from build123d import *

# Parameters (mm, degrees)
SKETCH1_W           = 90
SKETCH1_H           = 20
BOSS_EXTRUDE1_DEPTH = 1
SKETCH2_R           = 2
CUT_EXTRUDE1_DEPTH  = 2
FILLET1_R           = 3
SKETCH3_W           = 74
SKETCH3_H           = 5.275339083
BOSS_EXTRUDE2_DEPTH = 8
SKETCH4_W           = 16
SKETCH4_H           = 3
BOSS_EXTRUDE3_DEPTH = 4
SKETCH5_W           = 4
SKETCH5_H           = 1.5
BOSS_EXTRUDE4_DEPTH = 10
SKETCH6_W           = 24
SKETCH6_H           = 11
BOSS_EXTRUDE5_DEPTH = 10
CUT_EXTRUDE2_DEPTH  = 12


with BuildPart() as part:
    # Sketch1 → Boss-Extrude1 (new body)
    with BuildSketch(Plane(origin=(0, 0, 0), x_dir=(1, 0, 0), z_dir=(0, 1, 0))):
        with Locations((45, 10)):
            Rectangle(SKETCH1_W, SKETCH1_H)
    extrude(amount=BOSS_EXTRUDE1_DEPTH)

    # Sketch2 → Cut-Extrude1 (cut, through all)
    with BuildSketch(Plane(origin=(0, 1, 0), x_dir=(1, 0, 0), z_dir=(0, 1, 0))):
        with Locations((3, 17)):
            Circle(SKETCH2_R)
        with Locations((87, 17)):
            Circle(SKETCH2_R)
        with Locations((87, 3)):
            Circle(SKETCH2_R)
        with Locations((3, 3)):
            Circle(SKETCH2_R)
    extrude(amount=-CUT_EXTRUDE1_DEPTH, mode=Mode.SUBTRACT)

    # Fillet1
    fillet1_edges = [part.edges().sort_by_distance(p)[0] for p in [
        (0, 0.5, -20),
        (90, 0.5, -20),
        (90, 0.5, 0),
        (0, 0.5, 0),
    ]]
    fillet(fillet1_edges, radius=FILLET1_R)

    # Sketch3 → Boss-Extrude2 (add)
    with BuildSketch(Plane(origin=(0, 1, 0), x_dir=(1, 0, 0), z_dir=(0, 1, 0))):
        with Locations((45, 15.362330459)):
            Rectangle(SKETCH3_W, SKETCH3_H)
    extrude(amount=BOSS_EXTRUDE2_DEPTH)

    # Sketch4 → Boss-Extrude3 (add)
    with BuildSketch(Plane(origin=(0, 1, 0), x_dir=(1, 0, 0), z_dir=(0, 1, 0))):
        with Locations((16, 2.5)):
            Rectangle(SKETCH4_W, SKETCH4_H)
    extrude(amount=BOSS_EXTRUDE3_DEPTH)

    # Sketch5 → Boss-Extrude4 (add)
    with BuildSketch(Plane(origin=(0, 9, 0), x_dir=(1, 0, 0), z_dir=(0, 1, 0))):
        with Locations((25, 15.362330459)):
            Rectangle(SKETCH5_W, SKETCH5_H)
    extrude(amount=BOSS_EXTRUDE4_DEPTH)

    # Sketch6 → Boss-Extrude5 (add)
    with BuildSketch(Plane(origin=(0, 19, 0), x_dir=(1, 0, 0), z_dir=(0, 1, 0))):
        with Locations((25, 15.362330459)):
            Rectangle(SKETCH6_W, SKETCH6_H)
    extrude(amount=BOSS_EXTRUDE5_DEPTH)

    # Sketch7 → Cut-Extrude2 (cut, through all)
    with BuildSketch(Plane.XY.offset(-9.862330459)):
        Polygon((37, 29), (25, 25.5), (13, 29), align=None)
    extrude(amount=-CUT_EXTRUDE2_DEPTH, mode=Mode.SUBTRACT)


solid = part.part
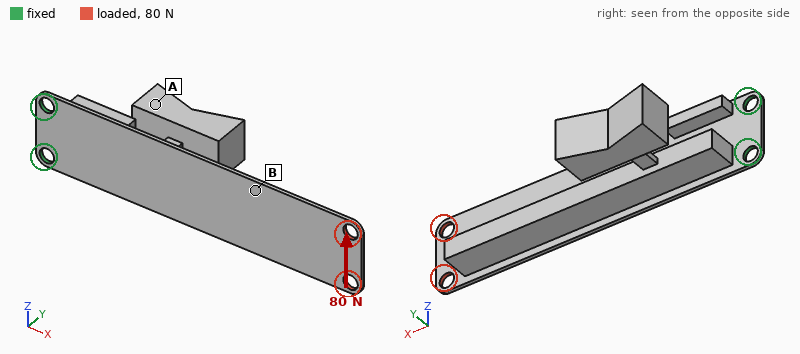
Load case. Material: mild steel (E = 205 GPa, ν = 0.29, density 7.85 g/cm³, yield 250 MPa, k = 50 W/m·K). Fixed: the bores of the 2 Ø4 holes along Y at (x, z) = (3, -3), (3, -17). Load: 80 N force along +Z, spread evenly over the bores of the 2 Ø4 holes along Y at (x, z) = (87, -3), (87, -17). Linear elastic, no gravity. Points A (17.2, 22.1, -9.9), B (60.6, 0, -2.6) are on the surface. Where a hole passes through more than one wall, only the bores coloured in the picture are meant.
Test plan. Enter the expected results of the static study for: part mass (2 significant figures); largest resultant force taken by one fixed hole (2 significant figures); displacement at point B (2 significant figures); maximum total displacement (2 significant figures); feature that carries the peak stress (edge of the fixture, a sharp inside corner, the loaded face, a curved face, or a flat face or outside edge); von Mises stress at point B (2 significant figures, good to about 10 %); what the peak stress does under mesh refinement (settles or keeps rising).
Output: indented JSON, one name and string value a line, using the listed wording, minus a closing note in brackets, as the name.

{
  "part mass": "57 g",
  "largest resultant force taken by one fixed hole": "450 N",
  "displacement at point B": "50 µm",
  "maximum total displacement": "96 µm",
  "feature that carries the peak stress": "edge of the fixture",
  "von Mises stress at point B": "20 MPa",
  "what the peak stress does under mesh refinement": "keeps rising"
}
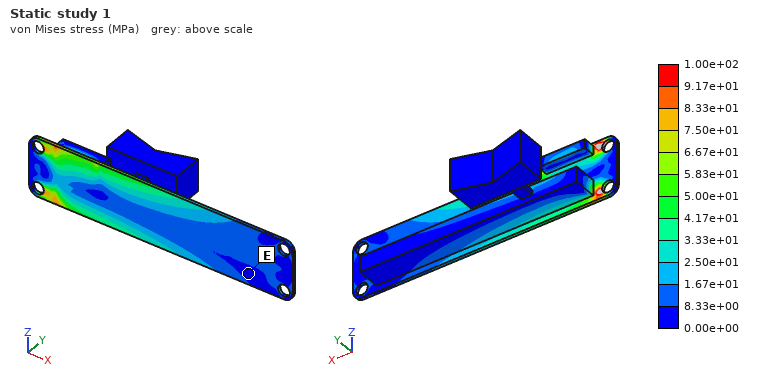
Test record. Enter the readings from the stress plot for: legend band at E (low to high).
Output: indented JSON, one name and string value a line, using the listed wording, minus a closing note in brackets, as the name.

{
  "legend band at E": "0.00e+00 to 8.33e+00 MPa"
}
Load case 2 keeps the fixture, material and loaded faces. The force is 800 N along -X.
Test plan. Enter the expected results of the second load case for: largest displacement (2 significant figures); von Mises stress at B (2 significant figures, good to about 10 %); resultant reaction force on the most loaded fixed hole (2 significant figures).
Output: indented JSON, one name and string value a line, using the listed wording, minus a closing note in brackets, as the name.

{
  "largest displacement": "89 µm",
  "von Mises stress at B": "42 MPa",
  "resultant reaction force on the most loaded fixed hole": "410 N"
}
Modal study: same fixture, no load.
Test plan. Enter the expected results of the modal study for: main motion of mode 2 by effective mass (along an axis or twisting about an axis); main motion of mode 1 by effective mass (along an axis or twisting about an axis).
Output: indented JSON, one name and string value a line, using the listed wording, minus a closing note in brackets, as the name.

{
  "main motion of mode 2 by effective mass": "along Z",
  "main motion of mode 1 by effective mass": "along Y"
}
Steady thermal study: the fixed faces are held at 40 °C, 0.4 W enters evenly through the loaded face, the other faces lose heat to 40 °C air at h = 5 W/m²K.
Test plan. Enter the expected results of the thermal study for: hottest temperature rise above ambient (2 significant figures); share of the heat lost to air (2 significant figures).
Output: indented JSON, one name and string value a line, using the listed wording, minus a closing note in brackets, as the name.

{
  "hottest temperature rise above ambient": "14 K",
  "share of the heat lost to air": "36 %"
}
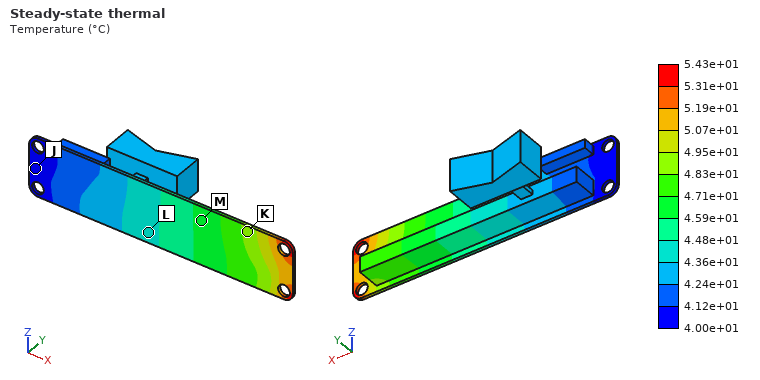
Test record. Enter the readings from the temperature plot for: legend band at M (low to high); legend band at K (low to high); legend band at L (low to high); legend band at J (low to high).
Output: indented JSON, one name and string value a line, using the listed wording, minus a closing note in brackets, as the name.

{
  "legend band at M": "4.59e+01 to 4.71e+01 °C",
  "legend band at K": "4.83e+01 to 4.95e+01 °C",
  "legend band at L": "4.36e+01 to 4.48e+01 °C",
  "legend band at J": "4.00e+01 to 4.12e+01 °C"
}
